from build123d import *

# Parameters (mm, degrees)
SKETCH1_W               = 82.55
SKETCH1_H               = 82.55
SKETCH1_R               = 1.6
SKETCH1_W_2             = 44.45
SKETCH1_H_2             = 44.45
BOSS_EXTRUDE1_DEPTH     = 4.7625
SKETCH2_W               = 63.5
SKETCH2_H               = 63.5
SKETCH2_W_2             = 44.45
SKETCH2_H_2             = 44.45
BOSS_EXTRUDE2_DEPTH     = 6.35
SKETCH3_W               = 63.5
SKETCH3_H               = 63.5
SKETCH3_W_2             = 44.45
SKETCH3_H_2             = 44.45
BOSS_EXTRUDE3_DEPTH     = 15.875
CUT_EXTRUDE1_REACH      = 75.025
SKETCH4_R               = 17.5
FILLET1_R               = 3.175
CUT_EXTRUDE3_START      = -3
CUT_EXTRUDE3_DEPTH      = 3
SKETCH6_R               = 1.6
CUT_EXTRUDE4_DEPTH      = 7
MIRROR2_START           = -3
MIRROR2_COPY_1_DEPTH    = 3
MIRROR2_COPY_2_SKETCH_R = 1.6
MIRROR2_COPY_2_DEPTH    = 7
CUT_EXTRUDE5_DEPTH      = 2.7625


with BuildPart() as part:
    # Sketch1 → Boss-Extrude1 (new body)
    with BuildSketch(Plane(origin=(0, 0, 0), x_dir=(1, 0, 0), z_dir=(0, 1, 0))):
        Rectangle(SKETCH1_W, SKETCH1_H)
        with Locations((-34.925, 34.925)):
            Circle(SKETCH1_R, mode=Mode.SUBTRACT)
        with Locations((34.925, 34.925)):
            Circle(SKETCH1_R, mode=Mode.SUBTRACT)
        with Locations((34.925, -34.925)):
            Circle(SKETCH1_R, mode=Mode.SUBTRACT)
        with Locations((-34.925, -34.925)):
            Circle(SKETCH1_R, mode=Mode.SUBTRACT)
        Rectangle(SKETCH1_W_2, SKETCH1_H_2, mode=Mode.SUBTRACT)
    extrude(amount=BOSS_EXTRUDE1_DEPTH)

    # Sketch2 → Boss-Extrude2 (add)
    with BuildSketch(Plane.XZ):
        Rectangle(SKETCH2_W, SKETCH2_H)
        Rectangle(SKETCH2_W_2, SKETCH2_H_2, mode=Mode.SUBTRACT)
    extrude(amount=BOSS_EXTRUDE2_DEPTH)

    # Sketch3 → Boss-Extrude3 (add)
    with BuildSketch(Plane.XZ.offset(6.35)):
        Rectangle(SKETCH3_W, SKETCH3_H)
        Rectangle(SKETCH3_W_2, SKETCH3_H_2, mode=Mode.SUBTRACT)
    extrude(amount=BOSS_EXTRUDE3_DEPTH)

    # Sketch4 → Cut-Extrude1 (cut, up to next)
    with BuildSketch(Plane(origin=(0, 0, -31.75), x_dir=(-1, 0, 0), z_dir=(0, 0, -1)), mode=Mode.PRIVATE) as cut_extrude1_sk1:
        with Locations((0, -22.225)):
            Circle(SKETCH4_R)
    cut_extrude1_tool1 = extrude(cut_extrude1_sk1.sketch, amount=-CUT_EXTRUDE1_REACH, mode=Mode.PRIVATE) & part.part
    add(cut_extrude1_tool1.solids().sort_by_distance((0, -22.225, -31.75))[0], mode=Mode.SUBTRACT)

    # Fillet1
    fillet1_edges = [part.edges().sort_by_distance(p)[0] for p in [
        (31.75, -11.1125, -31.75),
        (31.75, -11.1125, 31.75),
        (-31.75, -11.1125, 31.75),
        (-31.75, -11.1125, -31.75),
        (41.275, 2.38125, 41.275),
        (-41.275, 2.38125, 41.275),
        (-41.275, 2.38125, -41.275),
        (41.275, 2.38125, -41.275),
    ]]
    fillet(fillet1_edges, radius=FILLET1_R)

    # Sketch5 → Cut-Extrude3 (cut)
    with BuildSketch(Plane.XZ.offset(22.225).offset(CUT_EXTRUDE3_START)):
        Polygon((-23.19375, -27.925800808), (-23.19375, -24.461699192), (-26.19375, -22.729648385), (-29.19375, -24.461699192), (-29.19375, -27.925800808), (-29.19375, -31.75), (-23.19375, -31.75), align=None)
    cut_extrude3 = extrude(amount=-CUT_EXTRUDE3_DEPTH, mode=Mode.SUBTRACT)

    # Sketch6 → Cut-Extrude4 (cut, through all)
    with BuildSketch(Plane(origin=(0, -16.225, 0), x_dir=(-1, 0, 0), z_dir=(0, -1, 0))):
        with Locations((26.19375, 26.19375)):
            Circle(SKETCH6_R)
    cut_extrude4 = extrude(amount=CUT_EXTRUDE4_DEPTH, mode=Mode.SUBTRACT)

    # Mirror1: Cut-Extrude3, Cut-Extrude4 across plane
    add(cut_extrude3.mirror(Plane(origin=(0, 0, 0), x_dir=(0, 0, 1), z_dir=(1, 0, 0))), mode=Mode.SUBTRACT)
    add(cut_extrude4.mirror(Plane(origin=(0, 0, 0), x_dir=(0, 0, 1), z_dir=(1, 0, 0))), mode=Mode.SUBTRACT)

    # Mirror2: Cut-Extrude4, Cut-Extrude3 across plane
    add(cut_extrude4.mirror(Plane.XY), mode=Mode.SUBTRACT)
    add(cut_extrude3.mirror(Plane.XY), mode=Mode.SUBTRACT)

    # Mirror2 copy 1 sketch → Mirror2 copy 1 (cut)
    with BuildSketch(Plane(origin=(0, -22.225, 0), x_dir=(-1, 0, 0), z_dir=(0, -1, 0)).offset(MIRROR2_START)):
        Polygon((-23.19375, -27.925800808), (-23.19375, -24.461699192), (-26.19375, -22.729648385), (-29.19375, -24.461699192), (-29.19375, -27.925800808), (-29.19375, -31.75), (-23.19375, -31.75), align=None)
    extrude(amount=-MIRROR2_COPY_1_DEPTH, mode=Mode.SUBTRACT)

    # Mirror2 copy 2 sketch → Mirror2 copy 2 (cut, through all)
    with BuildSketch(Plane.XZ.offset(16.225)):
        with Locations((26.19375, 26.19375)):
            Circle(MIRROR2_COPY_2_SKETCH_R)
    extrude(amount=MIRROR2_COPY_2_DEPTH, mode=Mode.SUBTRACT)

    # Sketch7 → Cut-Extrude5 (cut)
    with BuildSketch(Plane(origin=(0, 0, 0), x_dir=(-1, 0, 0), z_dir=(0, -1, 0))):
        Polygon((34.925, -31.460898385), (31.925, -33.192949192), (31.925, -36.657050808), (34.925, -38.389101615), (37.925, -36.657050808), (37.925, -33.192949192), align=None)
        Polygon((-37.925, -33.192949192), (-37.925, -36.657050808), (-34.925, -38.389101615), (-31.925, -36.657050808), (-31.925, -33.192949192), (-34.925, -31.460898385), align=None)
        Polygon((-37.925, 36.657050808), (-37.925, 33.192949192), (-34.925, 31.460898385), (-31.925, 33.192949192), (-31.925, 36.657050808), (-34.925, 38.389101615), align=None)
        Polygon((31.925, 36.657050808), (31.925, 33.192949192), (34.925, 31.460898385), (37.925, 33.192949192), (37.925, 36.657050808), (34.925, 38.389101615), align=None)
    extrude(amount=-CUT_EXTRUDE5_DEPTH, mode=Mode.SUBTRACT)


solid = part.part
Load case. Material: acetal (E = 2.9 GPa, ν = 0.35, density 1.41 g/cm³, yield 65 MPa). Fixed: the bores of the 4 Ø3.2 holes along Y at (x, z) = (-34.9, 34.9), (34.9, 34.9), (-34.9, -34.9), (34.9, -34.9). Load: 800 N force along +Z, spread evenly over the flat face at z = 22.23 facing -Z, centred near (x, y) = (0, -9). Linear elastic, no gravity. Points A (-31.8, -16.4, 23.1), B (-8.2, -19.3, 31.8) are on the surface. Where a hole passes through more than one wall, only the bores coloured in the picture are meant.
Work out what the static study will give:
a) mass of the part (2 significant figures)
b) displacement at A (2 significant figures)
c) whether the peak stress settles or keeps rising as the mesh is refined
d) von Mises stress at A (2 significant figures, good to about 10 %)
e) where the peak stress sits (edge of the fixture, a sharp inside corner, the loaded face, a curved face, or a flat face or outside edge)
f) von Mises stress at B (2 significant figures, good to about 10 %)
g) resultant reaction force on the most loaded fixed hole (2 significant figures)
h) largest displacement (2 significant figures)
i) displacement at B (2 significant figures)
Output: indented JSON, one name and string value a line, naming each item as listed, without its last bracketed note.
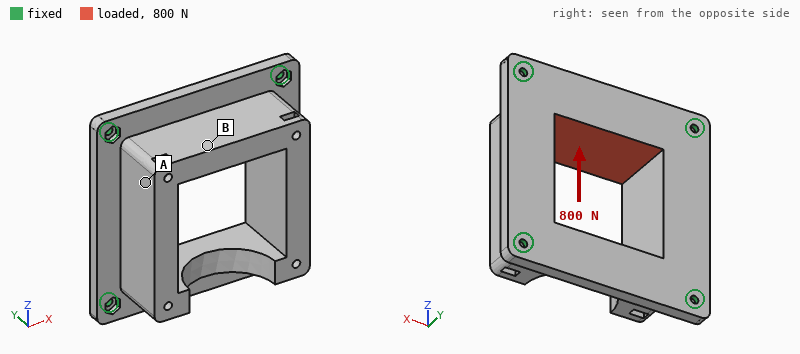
{
  "mass of the part": "89 g",
  "displacement at A": "0.037 mm",
  "whether the peak stress settles or keeps rising as the mesh is refined": "keeps rising",
  "von Mises stress at A": "2.2 MPa",
  "where the peak stress sits": "edge of the fixture",
  "von Mises stress at B": "5.7 MPa",
  "resultant reaction force on the most loaded fixed hole": "240 N",
  "largest displacement": "0.19 mm",
  "displacement at B": "0.16 mm"
}
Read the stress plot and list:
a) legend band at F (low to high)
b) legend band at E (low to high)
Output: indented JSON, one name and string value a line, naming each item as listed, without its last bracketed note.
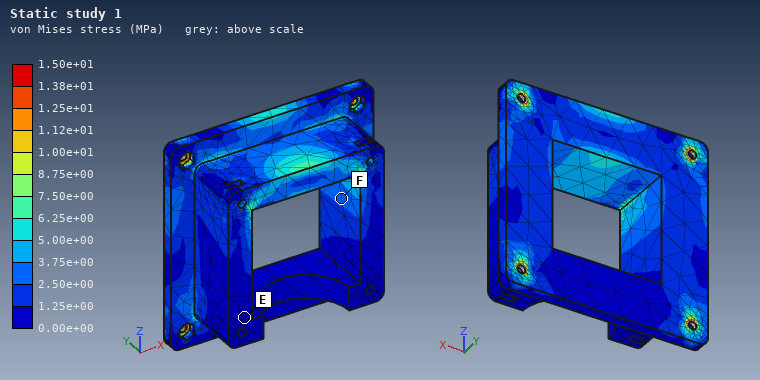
{
  "legend band at F": "2.50e+00 to 3.75e+00 MPa",
  "legend band at E": "0.00e+00 to 1.25e+00 MPa"
}
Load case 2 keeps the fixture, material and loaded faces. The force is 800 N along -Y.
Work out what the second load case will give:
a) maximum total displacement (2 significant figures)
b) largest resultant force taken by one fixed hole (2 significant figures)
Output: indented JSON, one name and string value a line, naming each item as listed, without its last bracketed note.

{
  "maximum total displacement": "0.23 mm",
  "largest resultant force taken by one fixed hole": "440 N"
}
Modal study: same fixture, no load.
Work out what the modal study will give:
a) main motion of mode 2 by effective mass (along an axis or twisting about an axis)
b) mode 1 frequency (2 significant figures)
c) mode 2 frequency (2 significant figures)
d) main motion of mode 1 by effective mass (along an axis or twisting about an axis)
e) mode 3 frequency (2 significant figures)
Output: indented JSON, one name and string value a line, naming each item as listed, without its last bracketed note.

{
  "main motion of mode 2 by effective mass": "along Y",
  "mode 1 frequency": "1300 Hz",
  "mode 2 frequency": "1600 Hz",
  "main motion of mode 1 by effective mass": "along Y",
  "mode 3 frequency": "1800 Hz"
}
